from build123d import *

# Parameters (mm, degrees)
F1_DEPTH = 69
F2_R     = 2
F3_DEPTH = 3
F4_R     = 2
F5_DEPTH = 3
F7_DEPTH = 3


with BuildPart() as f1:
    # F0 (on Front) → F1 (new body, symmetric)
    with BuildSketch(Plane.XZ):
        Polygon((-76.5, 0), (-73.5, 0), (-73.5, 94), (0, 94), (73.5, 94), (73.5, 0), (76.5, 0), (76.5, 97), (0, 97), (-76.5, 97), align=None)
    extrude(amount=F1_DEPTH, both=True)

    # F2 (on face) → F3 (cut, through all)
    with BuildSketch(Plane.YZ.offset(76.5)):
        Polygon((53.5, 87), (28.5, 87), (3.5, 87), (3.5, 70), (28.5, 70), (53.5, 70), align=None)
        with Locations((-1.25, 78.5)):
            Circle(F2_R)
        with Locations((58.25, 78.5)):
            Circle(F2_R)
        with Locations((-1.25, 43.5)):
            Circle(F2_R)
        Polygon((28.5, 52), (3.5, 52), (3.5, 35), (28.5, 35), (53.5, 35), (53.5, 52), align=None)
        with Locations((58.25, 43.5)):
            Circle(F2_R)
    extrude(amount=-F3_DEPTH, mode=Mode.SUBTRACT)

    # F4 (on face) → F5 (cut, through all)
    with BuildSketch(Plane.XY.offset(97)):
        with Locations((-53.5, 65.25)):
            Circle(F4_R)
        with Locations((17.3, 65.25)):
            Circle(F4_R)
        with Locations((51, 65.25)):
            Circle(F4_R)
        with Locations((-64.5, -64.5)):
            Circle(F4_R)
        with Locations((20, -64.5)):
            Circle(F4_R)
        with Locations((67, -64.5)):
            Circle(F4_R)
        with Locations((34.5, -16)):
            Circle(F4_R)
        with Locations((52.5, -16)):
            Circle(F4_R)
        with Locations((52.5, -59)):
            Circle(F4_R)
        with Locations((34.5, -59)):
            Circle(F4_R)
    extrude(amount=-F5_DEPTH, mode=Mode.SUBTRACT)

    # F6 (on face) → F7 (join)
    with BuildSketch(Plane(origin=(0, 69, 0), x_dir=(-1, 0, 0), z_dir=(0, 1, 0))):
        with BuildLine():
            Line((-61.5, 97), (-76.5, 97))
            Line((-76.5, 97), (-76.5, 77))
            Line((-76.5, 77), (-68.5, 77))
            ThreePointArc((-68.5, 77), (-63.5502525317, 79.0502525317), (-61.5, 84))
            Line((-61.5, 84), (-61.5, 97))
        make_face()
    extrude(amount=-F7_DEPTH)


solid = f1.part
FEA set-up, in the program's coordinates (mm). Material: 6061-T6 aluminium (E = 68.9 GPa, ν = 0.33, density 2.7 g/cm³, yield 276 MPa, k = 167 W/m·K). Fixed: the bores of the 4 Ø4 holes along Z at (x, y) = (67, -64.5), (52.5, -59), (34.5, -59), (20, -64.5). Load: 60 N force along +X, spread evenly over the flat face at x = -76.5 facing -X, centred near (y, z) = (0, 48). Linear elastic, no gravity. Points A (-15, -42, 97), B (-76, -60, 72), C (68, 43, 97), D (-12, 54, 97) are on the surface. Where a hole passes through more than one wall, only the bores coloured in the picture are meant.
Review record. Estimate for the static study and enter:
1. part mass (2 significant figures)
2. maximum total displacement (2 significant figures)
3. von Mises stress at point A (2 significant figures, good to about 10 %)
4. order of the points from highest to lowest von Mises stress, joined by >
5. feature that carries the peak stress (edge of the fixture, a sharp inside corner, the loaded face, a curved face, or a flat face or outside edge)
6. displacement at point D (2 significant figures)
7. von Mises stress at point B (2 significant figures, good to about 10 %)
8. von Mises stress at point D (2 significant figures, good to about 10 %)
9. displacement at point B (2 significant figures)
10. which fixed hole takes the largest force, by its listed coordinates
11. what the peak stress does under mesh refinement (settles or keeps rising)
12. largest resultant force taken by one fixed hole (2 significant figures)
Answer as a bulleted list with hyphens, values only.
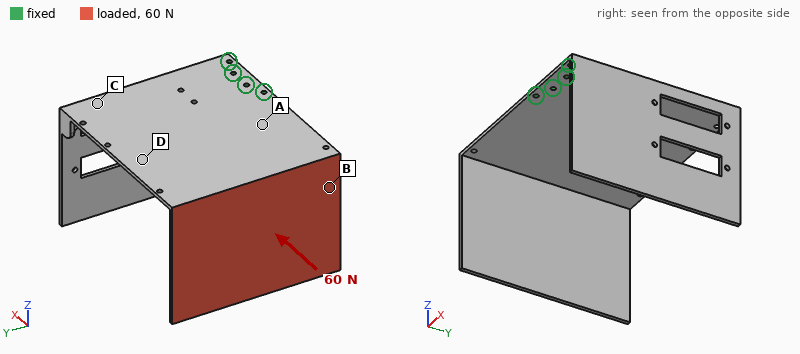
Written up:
- 370 g
- 2.2 mm
- 15 MPa
- A > D > B > C
- edge of the fixture
- 0.35 mm
- 7.2 MPa
- 11 MPa
- 0.99 mm
- (20, -64.5)
- keeps rising
- 88 N
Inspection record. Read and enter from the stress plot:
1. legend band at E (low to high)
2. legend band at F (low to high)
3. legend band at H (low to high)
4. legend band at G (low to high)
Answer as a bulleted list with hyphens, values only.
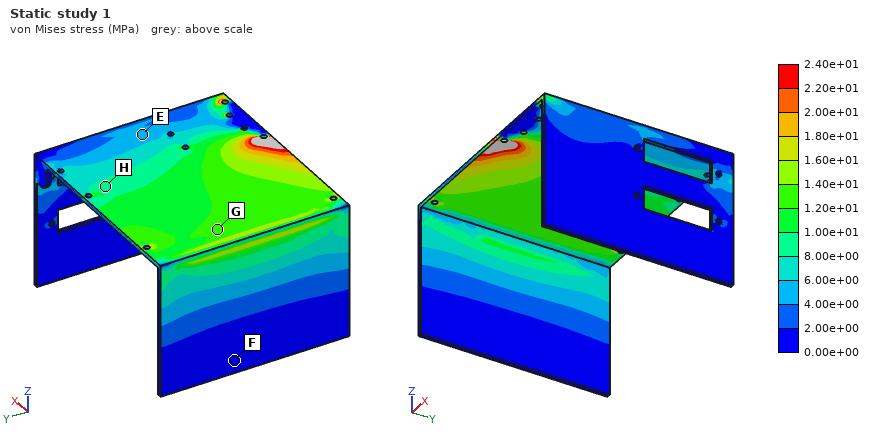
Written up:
- 4.00e+00 to 6.00e+00 MPa
- 0.00e+00 to 2.00e+00 MPa
- 8.00e+00 to 1.00e+01 MPa
- 1.20e+01 to 1.40e+01 MPa
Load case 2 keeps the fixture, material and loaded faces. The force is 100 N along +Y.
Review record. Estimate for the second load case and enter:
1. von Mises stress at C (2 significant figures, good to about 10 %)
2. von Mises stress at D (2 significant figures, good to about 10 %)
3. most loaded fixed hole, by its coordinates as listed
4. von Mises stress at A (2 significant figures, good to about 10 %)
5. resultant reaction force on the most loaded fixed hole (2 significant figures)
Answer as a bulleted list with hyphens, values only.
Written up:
- 8.6 MPa
- 14 MPa
- (20, -64.5)
- 19 MPa
- 280 N
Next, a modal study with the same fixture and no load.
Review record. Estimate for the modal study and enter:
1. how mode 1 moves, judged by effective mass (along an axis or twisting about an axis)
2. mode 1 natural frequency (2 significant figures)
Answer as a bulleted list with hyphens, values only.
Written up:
- along Z
- 61 Hz
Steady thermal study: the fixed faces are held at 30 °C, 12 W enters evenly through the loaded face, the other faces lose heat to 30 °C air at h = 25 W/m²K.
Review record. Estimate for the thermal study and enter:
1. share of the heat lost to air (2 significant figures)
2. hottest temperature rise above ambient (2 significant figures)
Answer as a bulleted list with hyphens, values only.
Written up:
- 78 %
- 14 K
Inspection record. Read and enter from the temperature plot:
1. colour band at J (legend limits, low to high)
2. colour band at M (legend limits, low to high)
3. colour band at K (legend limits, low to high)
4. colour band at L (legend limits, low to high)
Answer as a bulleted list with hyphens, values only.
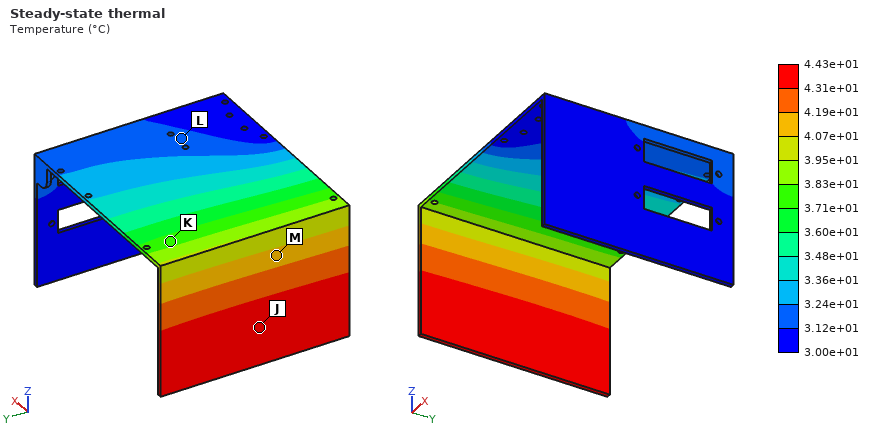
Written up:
- 4.31e+01 to 4.43e+01 °C
- 4.07e+01 to 4.19e+01 °C
- 3.71e+01 to 3.83e+01 °C
- 3.12e+01 to 3.24e+01 °C
